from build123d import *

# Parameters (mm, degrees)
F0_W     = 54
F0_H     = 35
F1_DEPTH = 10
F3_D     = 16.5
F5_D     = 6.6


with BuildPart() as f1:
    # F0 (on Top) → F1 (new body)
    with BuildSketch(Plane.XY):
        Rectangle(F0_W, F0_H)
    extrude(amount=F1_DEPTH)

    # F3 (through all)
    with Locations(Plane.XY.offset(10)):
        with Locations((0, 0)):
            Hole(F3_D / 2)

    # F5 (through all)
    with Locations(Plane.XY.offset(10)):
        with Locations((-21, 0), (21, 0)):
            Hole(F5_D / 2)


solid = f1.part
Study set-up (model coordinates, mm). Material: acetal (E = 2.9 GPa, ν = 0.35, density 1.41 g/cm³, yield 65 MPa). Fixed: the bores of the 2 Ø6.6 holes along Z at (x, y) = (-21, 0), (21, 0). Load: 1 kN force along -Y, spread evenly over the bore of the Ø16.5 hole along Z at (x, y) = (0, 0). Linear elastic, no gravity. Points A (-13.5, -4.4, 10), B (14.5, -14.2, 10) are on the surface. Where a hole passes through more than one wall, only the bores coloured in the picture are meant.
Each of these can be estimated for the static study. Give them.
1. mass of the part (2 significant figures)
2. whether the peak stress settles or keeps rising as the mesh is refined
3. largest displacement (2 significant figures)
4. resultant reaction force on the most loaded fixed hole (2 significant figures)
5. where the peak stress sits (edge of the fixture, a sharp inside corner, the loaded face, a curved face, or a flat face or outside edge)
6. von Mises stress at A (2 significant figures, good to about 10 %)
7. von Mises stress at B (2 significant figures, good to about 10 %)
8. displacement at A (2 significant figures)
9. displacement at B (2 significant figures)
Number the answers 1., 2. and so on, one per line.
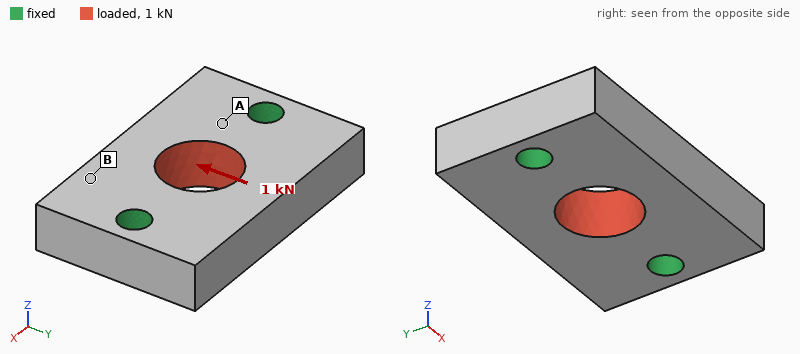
1. 23 g
2. keeps rising
3. 39 µm
4. 500 N
5. edge of the fixture
6. 3.6 MPa
7. 1.4 MPa
8. 15 µm
9. 17 µm
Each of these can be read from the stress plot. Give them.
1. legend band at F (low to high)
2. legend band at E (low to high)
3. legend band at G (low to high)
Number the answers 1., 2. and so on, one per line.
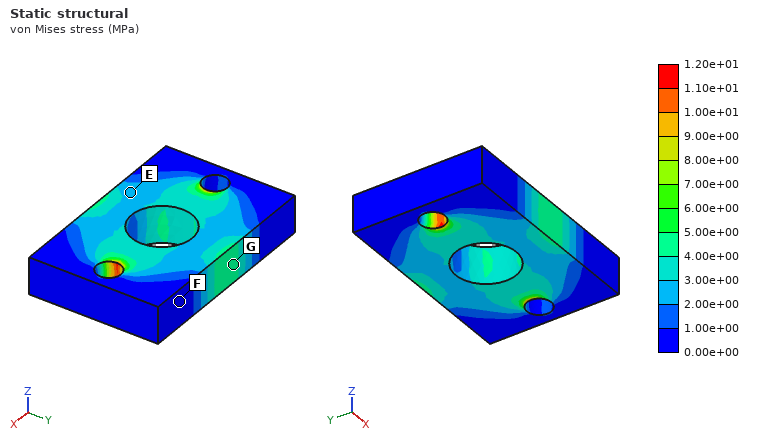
1. 0.00e+00 to 1.00e+00 MPa
2. 2.00e+00 to 3.00e+00 MPa
3. 4.00e+00 to 5.00e+00 MPa
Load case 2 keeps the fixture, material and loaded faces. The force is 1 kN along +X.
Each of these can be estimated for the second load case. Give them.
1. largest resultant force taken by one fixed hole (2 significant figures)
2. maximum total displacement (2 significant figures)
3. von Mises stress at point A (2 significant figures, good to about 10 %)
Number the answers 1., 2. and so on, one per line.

1. 500 N
2. 20 µm
3. 3.0 MPa
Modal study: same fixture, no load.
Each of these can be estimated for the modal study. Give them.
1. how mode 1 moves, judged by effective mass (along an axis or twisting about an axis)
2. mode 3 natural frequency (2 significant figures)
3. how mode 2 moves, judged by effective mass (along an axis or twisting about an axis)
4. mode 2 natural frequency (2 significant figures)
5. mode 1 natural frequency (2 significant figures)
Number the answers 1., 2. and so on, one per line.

1. twisting about X
2. 7500 Hz
3. along Z
4. 5100 Hz
5. 4600 Hz
